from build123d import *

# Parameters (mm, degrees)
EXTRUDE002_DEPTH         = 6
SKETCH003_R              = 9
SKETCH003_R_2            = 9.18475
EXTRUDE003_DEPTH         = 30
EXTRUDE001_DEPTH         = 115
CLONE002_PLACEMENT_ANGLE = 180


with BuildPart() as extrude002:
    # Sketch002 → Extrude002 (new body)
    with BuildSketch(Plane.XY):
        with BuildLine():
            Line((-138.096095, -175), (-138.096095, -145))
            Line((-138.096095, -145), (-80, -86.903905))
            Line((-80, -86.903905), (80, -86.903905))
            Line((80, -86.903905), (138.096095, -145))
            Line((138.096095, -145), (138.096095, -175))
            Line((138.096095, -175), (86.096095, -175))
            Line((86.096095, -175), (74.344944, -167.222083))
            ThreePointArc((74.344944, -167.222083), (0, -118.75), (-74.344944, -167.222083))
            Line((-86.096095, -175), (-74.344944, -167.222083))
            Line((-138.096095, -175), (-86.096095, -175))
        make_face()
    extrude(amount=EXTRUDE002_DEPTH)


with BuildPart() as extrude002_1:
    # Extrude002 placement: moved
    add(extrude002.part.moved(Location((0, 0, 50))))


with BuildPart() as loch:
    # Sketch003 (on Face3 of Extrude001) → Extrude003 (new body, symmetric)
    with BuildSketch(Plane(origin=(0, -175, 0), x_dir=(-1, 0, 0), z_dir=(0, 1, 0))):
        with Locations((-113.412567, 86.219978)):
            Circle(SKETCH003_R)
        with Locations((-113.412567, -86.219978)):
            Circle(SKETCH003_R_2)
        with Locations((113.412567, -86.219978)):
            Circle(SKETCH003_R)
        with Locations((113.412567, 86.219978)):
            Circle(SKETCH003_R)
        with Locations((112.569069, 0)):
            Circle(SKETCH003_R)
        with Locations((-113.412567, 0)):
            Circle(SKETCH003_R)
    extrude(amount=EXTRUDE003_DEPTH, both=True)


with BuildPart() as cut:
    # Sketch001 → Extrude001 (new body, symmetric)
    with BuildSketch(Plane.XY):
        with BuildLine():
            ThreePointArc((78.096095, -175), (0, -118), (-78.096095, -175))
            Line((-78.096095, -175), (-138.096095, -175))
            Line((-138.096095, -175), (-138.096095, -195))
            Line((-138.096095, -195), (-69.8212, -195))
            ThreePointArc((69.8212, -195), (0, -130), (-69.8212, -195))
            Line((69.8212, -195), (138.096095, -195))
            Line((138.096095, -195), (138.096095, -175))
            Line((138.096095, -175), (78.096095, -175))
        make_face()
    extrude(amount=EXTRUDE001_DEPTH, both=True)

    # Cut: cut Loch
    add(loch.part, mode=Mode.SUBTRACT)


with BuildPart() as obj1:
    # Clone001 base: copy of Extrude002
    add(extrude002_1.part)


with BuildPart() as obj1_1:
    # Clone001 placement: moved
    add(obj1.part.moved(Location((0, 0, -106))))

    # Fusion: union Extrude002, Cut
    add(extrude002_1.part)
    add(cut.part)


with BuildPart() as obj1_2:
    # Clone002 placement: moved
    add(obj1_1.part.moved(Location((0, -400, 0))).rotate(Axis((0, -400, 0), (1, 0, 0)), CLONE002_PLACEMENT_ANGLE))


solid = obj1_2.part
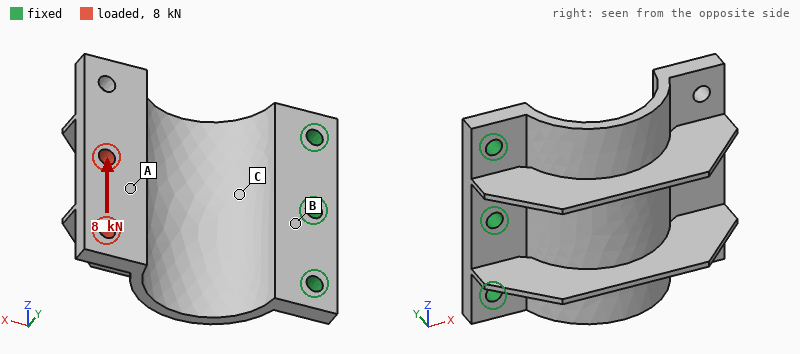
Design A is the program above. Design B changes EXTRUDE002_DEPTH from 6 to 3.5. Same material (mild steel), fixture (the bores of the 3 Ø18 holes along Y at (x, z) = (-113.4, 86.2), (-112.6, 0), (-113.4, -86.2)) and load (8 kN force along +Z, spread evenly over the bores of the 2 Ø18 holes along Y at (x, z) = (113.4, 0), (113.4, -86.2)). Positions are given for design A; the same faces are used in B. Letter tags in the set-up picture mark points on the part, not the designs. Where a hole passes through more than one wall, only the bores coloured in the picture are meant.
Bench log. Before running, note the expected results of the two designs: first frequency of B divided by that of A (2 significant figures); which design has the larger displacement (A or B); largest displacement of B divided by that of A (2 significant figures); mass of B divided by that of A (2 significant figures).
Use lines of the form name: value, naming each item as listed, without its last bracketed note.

first frequency of B divided by that of A: 0.90
which design has the larger displacement: B
largest displacement of B divided by that of A: 1.1
mass of B divided by that of A: 0.94
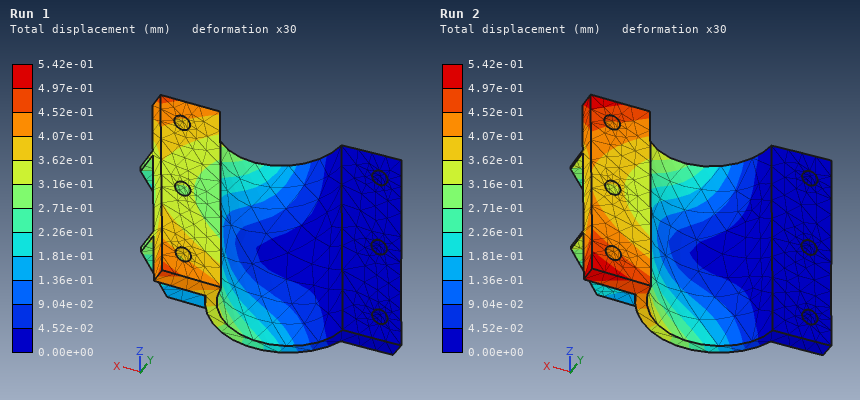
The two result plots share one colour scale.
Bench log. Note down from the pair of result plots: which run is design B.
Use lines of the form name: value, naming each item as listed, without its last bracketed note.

which run is design B: Run 2
